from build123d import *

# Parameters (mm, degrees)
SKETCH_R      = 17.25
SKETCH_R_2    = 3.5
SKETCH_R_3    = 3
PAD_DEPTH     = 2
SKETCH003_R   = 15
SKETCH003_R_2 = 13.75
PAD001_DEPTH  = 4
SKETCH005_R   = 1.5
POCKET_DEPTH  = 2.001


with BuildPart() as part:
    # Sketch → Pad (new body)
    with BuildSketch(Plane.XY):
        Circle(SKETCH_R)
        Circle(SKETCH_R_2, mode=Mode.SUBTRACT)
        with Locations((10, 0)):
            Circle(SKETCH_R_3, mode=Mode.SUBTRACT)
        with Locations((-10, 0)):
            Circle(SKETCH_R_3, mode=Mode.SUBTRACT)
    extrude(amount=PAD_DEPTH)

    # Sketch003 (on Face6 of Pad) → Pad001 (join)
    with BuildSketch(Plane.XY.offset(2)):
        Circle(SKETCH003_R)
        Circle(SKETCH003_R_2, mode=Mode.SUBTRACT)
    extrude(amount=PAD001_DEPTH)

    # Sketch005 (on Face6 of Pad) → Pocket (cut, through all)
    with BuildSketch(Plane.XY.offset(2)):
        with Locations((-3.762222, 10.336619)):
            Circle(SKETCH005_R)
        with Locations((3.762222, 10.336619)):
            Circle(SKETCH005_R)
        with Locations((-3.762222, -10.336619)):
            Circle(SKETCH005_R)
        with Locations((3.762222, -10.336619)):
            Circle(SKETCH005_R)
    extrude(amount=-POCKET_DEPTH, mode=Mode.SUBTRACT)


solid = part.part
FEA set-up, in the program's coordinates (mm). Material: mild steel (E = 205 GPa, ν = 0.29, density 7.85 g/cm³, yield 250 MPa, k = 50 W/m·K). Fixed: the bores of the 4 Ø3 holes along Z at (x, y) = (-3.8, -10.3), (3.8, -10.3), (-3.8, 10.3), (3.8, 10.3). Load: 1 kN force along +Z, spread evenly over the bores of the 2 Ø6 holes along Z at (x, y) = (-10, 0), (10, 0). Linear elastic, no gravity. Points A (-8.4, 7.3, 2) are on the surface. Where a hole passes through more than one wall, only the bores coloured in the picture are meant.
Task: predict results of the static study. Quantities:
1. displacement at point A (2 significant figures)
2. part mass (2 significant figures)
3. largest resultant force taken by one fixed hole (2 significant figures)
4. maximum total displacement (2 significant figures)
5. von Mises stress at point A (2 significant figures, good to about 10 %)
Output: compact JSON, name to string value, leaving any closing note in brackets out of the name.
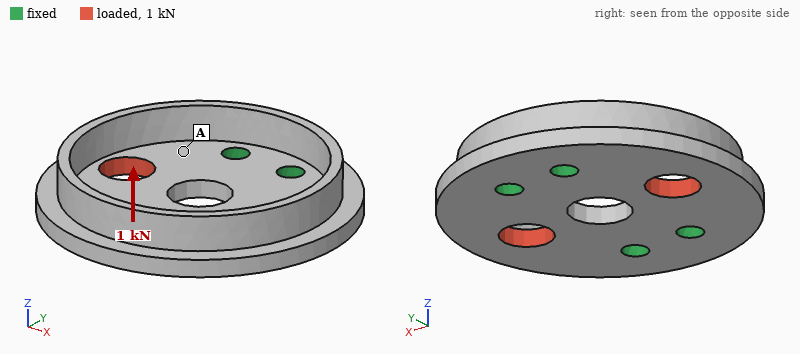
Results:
{"displacement at point A": "6.6 µm", "part mass": "16 g", "largest resultant force taken by one fixed hole": "270 N", "maximum total displacement": "22 µm", "von Mises stress at point A": "34 MPa"}
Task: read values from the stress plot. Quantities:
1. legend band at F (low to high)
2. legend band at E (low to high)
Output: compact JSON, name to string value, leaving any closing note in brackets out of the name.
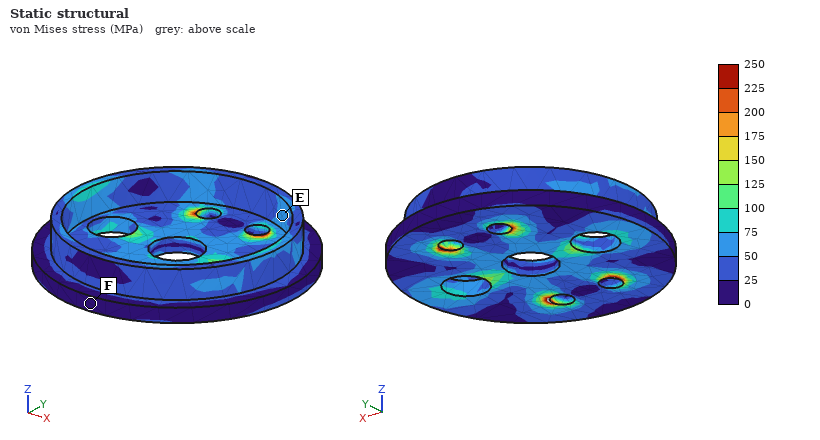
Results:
{"legend band at F": "0 to 25 MPa", "legend band at E": "50 to 75 MPa"}
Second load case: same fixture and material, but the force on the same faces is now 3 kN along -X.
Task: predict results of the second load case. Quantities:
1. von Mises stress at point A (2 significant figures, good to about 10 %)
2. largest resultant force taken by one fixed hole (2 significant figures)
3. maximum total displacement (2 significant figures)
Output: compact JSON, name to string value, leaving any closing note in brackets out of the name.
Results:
{"von Mises stress at point A": "47 MPa", "largest resultant force taken by one fixed hole": "760 N", "maximum total displacement": "4.6 µm"}
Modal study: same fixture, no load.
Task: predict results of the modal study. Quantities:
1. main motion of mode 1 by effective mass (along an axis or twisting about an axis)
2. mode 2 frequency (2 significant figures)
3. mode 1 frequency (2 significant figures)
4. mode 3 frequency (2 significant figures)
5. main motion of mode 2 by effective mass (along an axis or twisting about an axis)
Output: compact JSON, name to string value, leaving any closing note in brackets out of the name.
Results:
{"main motion of mode 1 by effective mass": "along Z", "mode 2 frequency": "13 kHz", "mode 1 frequency": "13 kHz", "mode 3 frequency": "25 kHz", "main motion of mode 2 by effective mass": "twisting about Y"}
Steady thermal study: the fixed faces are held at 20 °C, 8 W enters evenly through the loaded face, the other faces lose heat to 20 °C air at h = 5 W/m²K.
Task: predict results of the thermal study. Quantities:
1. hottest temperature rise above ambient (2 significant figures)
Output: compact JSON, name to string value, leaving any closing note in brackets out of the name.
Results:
{"hottest temperature rise above ambient": "18 K"}
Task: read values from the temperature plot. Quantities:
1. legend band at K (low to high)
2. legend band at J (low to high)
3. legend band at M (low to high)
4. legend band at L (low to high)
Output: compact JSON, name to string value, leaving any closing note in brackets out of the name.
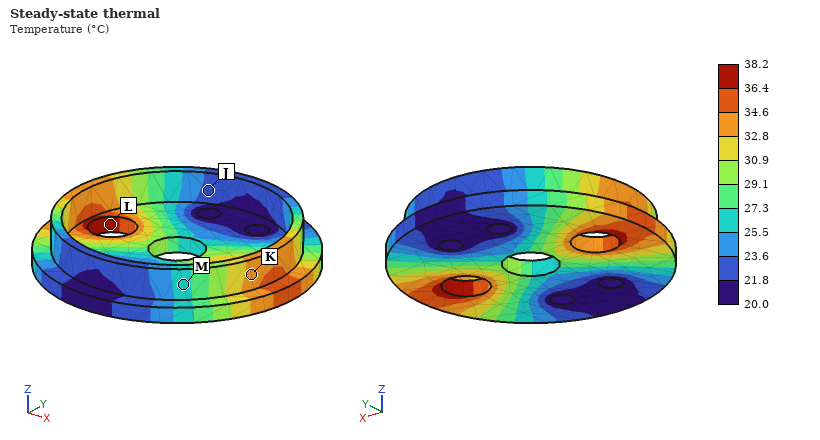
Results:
{"legend band at K": "32.8 to 34.6 °C", "legend band at J": "21.8 to 23.6 °C", "legend band at M": "25.5 to 27.3 °C", "legend band at L": "36.4 to 38.2 °C"}
